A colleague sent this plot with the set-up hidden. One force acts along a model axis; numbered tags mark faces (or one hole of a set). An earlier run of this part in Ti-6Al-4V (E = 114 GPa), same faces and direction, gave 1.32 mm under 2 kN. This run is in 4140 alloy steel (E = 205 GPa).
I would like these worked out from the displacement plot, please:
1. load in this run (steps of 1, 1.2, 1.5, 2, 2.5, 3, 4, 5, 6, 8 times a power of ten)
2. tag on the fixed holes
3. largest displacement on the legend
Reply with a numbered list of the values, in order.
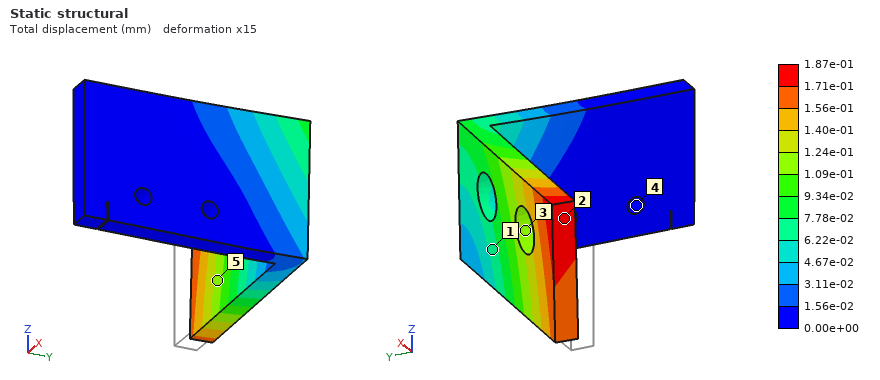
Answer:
1. 500 N
2. 4
3. 1.87e-01 mm
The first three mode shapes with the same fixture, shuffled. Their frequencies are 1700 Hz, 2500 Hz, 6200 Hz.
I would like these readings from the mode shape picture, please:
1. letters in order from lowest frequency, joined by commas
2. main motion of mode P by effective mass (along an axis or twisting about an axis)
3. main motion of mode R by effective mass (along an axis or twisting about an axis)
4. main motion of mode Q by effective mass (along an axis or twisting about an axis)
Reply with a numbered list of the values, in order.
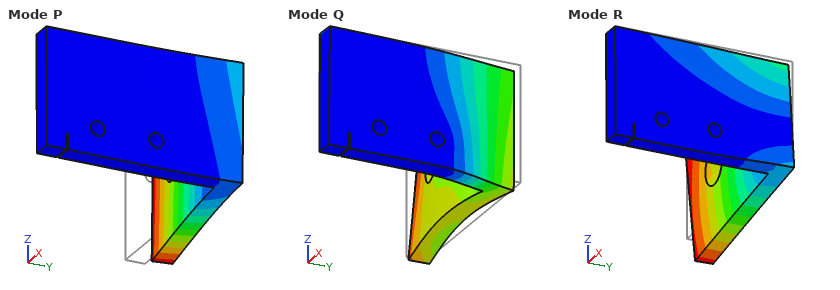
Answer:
1. P, R, Q
2. along Y
3. along Z
4. along X
